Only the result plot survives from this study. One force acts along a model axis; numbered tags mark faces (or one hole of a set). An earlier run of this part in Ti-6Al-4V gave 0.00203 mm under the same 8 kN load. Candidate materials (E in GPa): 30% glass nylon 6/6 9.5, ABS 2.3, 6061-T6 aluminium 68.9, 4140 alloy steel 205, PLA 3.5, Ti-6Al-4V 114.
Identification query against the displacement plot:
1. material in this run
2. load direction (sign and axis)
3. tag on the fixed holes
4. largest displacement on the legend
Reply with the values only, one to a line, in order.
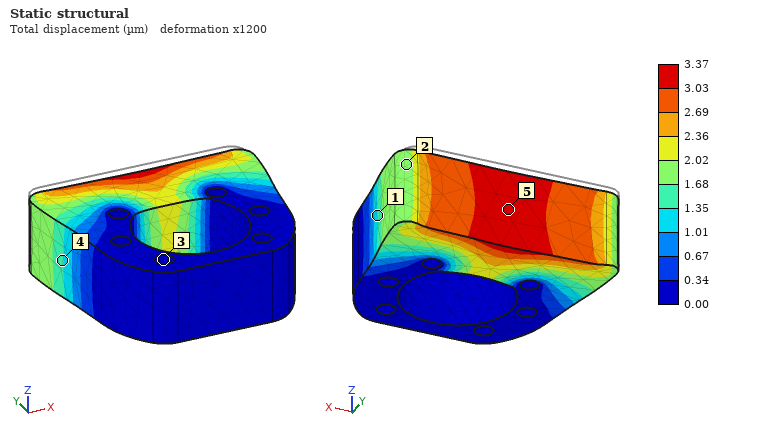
6061-T6 aluminium
-Y
3
3.37 µm
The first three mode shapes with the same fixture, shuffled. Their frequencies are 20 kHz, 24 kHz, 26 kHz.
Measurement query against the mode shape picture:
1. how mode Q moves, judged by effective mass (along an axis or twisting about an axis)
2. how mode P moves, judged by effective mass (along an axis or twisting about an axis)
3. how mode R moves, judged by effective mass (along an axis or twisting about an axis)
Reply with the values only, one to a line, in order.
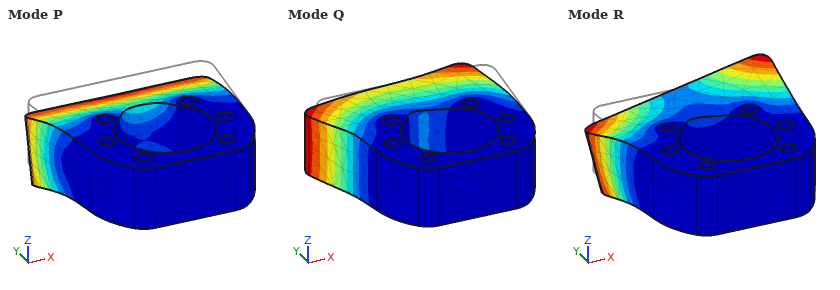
along X
along Z
twisting about Y
